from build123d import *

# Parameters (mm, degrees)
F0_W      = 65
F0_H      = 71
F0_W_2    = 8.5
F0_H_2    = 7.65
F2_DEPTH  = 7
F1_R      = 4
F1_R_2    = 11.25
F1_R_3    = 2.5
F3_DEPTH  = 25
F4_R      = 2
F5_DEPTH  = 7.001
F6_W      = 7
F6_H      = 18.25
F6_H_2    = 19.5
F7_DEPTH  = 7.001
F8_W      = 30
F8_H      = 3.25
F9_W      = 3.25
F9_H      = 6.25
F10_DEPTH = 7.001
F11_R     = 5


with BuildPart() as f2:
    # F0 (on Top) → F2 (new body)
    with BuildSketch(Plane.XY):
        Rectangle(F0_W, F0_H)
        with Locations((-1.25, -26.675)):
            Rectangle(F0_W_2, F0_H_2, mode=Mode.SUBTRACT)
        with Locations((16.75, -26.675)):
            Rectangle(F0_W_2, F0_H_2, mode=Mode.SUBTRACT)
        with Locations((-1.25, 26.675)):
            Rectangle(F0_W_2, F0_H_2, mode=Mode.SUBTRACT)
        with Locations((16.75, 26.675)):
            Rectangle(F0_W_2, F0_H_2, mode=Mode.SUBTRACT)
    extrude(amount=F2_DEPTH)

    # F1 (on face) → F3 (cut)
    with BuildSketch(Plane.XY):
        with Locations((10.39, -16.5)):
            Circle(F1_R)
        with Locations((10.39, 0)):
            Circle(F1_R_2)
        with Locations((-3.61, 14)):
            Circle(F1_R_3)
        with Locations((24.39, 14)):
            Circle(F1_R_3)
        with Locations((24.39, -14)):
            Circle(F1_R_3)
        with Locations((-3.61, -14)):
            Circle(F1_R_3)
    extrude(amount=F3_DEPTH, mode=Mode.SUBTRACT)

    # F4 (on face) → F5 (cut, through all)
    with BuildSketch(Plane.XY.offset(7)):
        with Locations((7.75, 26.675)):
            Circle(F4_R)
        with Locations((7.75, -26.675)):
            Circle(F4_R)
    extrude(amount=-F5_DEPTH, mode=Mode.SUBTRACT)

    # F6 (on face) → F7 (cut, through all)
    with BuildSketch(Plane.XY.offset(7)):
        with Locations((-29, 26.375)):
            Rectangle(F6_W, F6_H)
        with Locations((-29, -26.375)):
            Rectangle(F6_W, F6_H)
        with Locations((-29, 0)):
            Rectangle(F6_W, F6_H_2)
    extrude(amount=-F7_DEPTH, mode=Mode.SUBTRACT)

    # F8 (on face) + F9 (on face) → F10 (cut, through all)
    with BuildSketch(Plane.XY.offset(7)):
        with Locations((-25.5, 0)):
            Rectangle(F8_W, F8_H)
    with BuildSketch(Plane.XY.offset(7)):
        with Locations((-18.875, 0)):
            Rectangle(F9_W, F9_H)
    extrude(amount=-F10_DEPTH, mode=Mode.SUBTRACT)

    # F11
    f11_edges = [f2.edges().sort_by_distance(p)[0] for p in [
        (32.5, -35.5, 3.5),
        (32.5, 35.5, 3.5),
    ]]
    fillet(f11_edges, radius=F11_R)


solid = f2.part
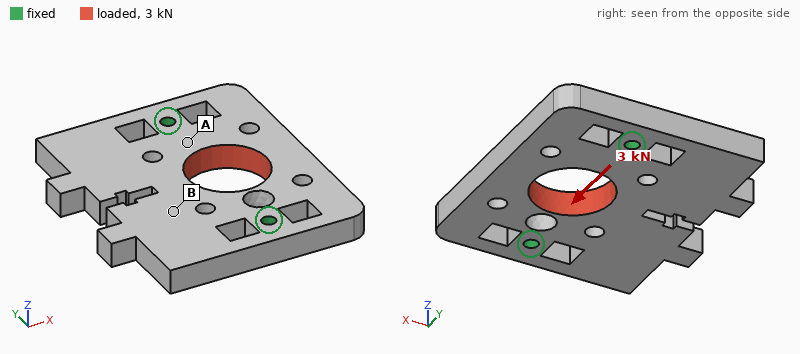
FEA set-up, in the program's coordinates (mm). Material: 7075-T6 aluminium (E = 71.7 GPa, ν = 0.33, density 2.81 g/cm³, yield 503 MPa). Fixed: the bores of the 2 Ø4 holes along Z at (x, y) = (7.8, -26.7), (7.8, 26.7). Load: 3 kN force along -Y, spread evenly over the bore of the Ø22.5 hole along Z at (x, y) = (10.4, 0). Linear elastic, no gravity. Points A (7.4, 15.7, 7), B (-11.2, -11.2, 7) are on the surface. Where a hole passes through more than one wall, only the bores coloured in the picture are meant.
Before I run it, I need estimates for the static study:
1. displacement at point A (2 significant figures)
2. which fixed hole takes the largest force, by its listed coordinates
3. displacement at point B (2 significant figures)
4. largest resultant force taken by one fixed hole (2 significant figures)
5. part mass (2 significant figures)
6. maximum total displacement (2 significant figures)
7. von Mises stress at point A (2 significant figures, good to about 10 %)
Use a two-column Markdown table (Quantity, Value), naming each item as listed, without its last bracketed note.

| Quantity | Value |
|---|---|
| displacement at point A | 2.4 µm |
| which fixed hole takes the largest force, by its listed coordinates | (7.8, 26.7) |
| displacement at point B | 3.5 µm |
| largest resultant force taken by one fixed hole | 1.7 kN |
| part mass | 66 g |
| maximum total displacement | 9.7 µm |
| von Mises stress at point A | 13 MPa |
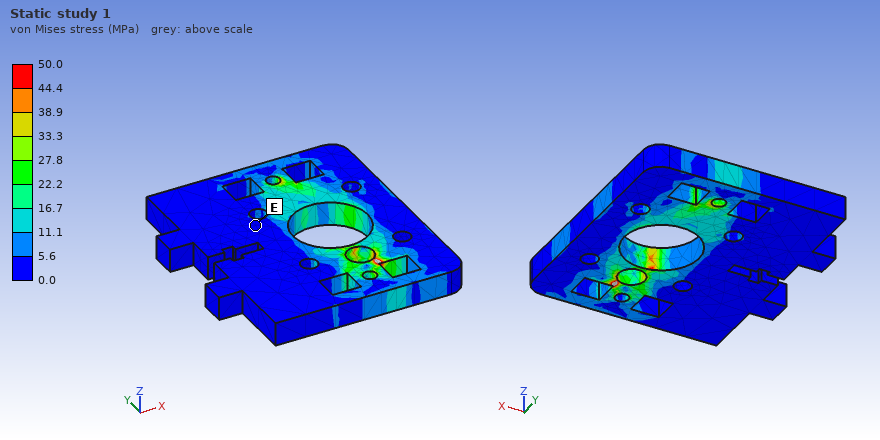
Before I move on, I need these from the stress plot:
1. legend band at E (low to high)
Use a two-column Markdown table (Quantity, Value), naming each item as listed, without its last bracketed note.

| Quantity | Value |
|---|---|
| legend band at E | 0.0 to 5.6 MPa |
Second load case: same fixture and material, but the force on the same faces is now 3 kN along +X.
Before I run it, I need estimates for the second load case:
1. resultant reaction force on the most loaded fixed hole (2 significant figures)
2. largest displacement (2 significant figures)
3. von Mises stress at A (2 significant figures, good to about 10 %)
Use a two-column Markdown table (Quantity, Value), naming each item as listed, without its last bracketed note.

| Quantity | Value |
|---|---|
| resultant reaction force on the most loaded fixed hole | 1.5 kN |
| largest displacement | 14 µm |
| von Mises stress at A | 10 MPa |
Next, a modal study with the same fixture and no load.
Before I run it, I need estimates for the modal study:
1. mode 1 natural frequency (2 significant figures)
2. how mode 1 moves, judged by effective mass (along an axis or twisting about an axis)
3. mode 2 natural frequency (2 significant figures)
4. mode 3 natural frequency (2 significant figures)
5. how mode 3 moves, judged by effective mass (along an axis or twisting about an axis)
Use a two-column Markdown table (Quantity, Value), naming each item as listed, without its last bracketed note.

| Quantity | Value |
|---|---|
| mode 1 natural frequency | 2600 Hz |
| how mode 1 moves, judged by effective mass | along Z |
| mode 2 natural frequency | 4400 Hz |
| mode 3 natural frequency | 4900 Hz |
| how mode 3 moves, judged by effective mass | along Z |
